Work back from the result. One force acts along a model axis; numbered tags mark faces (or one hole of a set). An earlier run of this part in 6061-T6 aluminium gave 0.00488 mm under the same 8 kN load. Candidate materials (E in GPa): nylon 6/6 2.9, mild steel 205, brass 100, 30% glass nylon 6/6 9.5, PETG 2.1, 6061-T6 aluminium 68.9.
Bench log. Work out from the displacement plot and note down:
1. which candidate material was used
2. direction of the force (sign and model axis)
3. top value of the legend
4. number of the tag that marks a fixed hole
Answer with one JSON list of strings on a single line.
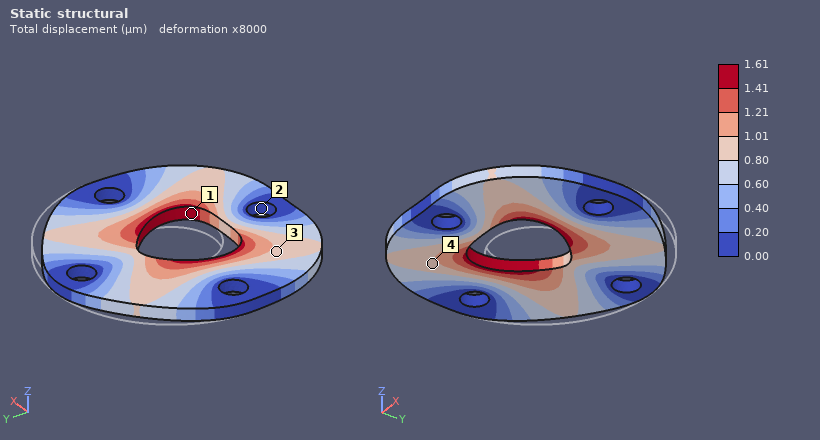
["mild steel", "-Y", "1.61 µm", "2"]
